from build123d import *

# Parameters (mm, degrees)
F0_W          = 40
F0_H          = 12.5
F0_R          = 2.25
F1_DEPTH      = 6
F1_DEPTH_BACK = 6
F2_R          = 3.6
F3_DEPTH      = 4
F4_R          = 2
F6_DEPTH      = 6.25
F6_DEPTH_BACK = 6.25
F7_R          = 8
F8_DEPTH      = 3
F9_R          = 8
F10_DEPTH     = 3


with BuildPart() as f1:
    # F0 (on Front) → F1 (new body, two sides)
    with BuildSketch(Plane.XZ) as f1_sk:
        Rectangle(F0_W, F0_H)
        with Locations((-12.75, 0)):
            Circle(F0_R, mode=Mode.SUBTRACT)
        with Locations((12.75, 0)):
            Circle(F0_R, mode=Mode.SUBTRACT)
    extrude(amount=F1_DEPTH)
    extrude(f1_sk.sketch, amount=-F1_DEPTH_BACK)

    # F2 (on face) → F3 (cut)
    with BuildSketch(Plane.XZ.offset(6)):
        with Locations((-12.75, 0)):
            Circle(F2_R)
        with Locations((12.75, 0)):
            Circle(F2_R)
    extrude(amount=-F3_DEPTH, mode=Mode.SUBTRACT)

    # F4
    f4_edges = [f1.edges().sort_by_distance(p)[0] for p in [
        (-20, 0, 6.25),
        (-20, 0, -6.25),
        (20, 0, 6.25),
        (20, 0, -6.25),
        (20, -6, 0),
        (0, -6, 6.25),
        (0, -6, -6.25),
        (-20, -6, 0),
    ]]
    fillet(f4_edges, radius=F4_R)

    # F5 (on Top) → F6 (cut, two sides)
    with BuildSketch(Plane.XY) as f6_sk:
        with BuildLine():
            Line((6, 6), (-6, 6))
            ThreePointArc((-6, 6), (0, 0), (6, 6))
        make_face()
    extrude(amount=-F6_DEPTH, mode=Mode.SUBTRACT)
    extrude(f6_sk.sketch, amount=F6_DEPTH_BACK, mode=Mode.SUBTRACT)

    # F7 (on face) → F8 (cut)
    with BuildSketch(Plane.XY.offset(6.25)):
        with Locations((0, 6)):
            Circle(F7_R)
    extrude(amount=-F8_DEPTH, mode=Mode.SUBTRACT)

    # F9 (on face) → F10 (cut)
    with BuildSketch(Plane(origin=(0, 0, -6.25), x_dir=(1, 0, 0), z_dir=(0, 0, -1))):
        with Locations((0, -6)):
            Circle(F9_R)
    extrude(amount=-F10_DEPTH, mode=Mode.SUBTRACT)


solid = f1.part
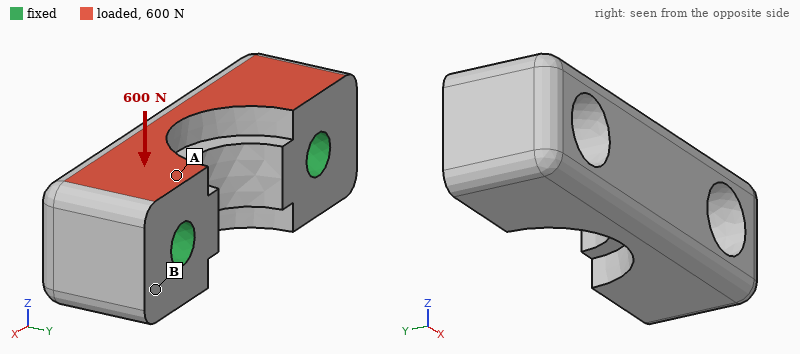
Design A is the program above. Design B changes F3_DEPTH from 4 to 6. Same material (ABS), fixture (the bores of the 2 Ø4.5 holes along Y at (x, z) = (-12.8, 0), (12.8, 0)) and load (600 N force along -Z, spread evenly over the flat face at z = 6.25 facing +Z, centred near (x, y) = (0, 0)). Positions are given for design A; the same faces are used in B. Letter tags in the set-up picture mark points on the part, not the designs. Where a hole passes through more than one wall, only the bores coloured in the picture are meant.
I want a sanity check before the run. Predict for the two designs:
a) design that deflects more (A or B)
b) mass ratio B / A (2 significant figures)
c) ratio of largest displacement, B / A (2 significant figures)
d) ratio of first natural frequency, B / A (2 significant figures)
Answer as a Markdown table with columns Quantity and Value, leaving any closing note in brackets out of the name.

| Quantity | Value |
|---|---|
| design that deflects more | B |
| mass ratio B / A | 0.98 |
| ratio of largest displacement, B / A | 1.8 |
| ratio of first natural frequency, B / A | 0.78 |
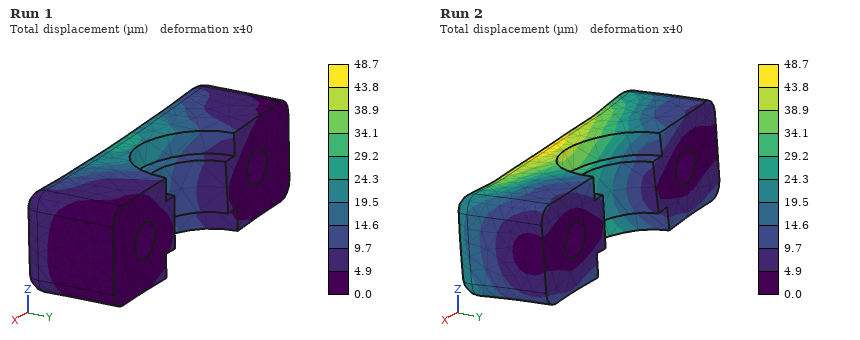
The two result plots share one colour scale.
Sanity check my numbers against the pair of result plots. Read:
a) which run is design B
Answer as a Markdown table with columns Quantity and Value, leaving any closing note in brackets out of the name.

| Quantity | Value |
|---|---|
| which run is design B | Run 2 |
